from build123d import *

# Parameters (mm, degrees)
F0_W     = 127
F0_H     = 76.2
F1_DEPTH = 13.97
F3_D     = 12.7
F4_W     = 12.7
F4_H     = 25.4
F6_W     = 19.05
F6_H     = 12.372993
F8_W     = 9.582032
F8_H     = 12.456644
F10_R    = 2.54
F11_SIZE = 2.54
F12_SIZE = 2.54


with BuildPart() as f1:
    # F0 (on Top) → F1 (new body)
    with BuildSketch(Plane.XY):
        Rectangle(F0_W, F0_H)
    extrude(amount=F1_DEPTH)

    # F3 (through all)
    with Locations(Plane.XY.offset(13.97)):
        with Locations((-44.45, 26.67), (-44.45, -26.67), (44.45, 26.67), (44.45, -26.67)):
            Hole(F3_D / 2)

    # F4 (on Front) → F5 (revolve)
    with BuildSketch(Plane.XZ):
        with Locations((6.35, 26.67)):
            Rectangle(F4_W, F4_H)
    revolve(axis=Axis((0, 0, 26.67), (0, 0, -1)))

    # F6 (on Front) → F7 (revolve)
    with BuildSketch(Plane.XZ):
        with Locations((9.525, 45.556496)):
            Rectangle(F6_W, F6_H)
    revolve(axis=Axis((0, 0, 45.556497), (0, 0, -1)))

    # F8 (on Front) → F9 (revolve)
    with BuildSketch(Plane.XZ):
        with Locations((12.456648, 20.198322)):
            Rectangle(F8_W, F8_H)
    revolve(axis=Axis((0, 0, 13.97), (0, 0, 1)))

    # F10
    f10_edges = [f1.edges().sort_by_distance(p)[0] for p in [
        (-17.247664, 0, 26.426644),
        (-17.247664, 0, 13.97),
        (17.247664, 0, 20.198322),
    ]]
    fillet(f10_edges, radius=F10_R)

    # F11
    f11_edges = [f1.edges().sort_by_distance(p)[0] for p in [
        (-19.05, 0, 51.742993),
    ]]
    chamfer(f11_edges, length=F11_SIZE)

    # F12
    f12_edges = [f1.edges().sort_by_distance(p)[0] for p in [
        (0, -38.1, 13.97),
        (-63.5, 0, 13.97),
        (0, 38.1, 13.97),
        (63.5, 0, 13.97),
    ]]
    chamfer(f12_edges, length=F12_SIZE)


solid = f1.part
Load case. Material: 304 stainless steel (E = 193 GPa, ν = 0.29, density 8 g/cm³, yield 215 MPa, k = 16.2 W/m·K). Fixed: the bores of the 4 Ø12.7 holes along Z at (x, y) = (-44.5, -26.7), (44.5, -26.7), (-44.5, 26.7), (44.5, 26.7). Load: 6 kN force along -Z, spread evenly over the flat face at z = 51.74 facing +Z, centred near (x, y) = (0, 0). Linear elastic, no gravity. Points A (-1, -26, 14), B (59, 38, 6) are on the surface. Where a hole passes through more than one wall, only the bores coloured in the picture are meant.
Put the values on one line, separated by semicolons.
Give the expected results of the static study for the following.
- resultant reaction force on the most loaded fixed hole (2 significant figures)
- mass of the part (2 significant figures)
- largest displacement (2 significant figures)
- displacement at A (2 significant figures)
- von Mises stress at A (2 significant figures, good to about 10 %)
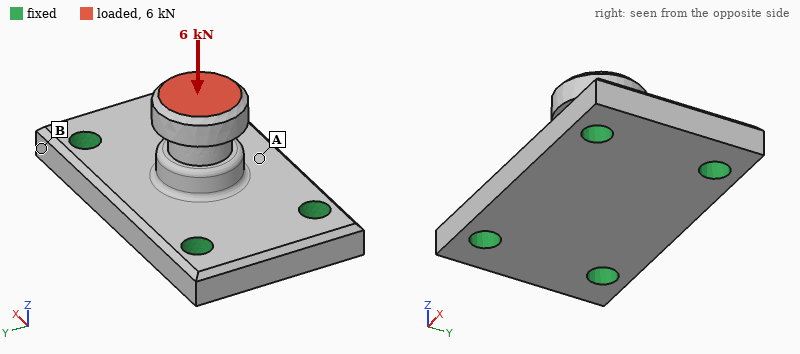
1.5 kN; 1.3 kg; 7.7 µm; 4.9 µm; 11 MPa
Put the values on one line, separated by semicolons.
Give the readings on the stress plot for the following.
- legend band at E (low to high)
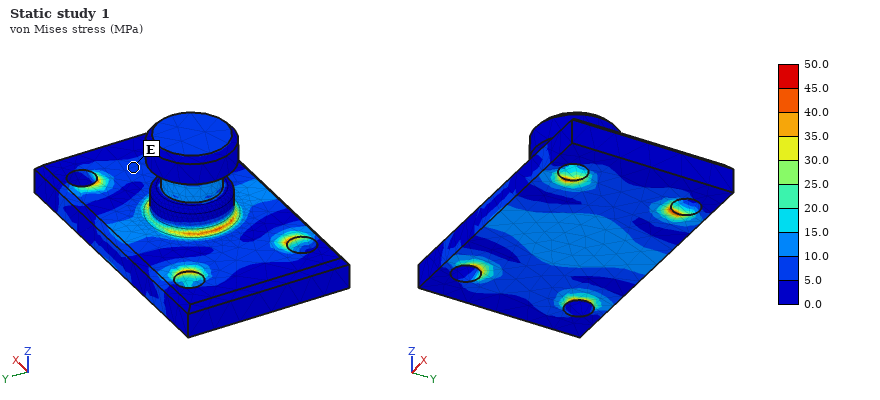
5.0 to 10.0 MPa
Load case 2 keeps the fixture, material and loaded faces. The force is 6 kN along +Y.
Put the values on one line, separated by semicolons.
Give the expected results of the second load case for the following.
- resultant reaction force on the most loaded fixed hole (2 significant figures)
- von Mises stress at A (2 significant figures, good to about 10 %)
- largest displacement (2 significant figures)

3.2 kN; 23 MPa; 49 µm
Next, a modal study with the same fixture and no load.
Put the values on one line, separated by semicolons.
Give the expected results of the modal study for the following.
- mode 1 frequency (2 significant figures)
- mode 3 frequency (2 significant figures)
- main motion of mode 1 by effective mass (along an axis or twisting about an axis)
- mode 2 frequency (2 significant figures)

5500 Hz; 6700 Hz; along Y; 6500 Hz
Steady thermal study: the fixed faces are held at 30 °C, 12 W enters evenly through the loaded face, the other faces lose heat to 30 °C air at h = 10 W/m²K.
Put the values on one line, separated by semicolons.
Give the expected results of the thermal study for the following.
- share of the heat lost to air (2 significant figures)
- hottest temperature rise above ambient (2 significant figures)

21 %; 52 K
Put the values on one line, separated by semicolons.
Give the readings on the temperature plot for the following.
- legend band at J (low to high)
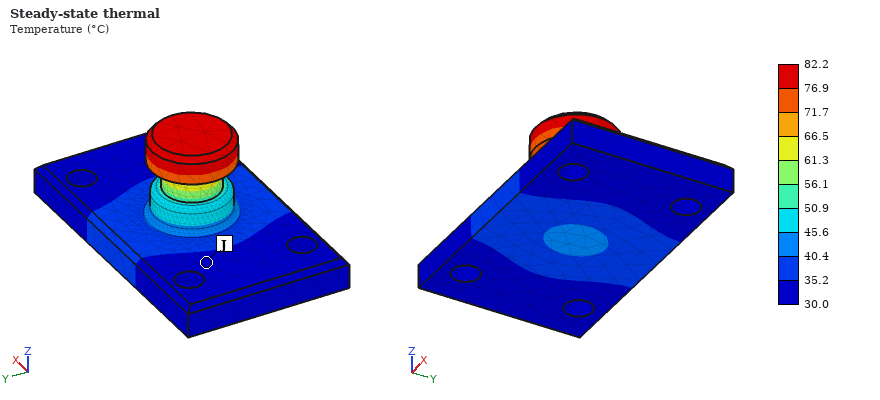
30.0 to 35.2 °C
